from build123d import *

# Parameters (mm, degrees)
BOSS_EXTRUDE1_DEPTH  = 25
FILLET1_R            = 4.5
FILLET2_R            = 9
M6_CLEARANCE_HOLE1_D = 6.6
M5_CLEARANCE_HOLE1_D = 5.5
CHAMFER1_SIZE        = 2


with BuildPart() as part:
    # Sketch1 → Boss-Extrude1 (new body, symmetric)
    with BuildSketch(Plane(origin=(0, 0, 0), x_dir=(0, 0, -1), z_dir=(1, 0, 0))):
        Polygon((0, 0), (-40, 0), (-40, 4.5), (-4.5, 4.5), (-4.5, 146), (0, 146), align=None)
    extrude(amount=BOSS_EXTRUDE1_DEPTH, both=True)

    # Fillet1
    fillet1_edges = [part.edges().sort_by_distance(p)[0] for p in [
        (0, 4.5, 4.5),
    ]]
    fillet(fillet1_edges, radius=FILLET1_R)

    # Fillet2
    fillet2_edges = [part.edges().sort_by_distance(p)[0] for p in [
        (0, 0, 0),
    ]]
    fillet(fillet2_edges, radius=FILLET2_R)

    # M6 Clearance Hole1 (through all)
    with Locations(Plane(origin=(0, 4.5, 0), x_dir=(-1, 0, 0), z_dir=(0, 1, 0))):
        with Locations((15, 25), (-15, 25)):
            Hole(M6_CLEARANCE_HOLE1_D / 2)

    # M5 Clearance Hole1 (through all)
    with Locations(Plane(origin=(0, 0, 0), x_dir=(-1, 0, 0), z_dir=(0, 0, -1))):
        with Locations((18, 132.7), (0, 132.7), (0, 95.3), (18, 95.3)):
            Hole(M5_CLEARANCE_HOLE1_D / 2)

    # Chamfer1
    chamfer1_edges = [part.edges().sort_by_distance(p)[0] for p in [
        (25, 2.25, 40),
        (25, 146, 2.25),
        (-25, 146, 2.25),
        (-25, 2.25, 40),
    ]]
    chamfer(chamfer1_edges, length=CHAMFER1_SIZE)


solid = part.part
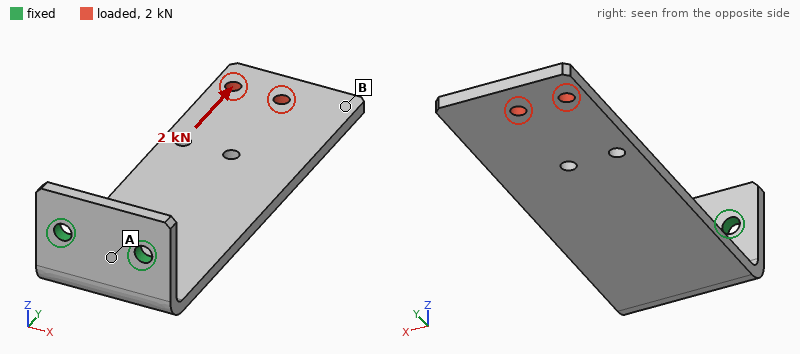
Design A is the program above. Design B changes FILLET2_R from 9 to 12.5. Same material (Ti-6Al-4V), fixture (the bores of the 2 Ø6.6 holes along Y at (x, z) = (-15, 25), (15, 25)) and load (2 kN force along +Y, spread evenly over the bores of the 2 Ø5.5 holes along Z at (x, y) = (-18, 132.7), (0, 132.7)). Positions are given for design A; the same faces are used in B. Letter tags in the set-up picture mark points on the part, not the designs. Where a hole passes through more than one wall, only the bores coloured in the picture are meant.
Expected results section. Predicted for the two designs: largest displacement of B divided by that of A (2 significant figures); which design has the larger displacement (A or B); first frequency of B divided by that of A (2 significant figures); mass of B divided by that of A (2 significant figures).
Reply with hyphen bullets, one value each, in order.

- 1.2
- B
- 0.89
- 0.98
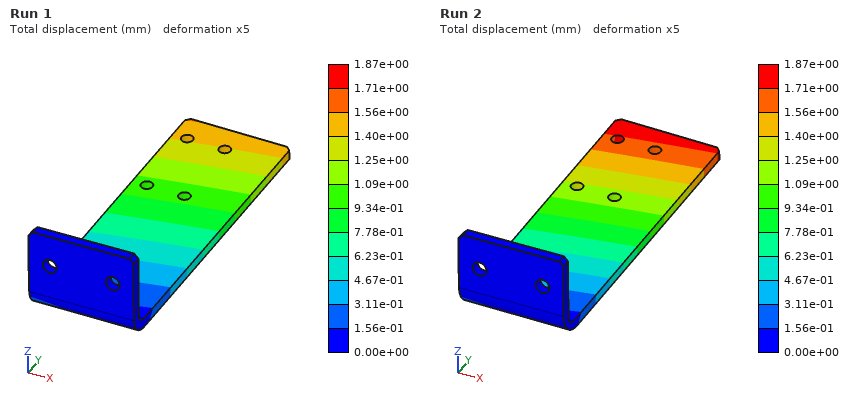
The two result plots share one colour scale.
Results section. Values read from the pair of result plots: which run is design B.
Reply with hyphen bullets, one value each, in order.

- Run 2
